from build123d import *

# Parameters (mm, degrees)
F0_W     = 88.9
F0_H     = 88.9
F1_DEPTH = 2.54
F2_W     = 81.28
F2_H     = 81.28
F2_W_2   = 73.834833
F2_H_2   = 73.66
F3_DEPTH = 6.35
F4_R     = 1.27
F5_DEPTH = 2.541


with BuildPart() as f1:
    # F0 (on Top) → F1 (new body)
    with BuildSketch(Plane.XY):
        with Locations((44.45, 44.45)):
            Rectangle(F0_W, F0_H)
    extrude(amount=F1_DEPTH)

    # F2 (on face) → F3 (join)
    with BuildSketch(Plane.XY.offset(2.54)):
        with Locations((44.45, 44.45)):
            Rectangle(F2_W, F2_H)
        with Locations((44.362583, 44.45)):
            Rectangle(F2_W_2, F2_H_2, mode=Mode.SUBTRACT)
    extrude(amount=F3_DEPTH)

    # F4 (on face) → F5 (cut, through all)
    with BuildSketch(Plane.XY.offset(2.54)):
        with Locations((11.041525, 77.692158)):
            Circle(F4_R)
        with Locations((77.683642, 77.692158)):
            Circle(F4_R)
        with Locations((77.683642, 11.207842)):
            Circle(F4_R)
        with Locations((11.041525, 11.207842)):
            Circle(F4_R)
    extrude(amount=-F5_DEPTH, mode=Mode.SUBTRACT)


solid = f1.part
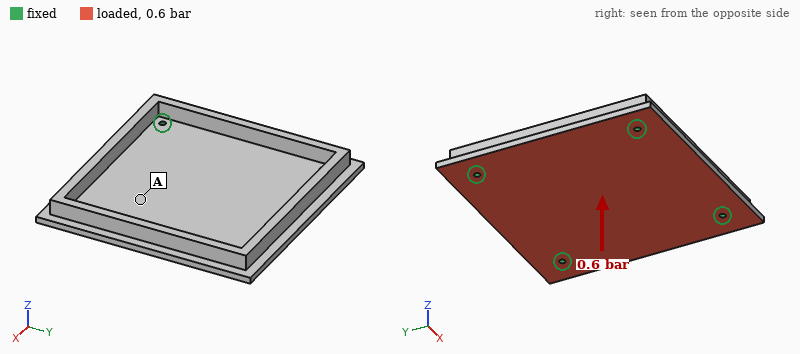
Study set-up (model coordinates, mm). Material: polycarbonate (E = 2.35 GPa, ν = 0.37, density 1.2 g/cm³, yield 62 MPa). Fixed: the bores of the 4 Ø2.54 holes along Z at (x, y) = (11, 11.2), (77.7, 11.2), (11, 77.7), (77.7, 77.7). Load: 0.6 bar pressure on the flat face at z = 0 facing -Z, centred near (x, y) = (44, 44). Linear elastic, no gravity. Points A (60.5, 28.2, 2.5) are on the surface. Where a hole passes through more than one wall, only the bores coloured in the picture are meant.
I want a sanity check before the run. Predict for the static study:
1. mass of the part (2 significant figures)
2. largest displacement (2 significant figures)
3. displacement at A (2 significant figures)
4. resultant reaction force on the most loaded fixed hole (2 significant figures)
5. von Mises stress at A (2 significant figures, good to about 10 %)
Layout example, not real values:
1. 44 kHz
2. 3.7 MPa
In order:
1. 33 g
2. 1.5 mm
3. 0.92 mm
4. 130 N
5. 6.2 MPa
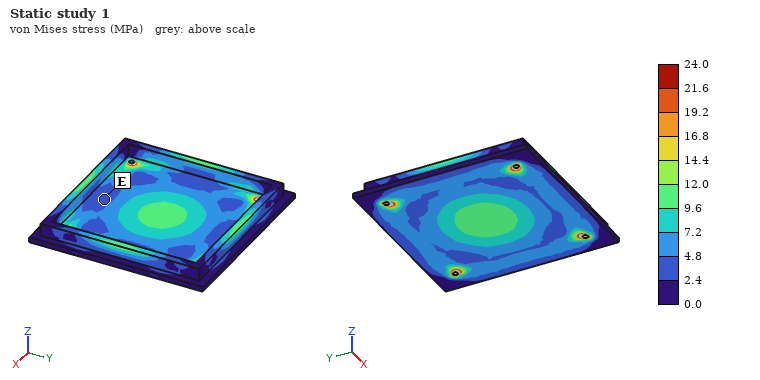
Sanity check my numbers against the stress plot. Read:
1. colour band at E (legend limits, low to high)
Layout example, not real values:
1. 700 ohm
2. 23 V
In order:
1. 2.4 to 4.8 MPa
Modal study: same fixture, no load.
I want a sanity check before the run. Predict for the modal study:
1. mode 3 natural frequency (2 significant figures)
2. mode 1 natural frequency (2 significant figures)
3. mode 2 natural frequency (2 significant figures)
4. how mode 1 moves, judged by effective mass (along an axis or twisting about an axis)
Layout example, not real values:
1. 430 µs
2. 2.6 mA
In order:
1. 1300 Hz
2. 720 Hz
3. 1300 Hz
4. along Z
